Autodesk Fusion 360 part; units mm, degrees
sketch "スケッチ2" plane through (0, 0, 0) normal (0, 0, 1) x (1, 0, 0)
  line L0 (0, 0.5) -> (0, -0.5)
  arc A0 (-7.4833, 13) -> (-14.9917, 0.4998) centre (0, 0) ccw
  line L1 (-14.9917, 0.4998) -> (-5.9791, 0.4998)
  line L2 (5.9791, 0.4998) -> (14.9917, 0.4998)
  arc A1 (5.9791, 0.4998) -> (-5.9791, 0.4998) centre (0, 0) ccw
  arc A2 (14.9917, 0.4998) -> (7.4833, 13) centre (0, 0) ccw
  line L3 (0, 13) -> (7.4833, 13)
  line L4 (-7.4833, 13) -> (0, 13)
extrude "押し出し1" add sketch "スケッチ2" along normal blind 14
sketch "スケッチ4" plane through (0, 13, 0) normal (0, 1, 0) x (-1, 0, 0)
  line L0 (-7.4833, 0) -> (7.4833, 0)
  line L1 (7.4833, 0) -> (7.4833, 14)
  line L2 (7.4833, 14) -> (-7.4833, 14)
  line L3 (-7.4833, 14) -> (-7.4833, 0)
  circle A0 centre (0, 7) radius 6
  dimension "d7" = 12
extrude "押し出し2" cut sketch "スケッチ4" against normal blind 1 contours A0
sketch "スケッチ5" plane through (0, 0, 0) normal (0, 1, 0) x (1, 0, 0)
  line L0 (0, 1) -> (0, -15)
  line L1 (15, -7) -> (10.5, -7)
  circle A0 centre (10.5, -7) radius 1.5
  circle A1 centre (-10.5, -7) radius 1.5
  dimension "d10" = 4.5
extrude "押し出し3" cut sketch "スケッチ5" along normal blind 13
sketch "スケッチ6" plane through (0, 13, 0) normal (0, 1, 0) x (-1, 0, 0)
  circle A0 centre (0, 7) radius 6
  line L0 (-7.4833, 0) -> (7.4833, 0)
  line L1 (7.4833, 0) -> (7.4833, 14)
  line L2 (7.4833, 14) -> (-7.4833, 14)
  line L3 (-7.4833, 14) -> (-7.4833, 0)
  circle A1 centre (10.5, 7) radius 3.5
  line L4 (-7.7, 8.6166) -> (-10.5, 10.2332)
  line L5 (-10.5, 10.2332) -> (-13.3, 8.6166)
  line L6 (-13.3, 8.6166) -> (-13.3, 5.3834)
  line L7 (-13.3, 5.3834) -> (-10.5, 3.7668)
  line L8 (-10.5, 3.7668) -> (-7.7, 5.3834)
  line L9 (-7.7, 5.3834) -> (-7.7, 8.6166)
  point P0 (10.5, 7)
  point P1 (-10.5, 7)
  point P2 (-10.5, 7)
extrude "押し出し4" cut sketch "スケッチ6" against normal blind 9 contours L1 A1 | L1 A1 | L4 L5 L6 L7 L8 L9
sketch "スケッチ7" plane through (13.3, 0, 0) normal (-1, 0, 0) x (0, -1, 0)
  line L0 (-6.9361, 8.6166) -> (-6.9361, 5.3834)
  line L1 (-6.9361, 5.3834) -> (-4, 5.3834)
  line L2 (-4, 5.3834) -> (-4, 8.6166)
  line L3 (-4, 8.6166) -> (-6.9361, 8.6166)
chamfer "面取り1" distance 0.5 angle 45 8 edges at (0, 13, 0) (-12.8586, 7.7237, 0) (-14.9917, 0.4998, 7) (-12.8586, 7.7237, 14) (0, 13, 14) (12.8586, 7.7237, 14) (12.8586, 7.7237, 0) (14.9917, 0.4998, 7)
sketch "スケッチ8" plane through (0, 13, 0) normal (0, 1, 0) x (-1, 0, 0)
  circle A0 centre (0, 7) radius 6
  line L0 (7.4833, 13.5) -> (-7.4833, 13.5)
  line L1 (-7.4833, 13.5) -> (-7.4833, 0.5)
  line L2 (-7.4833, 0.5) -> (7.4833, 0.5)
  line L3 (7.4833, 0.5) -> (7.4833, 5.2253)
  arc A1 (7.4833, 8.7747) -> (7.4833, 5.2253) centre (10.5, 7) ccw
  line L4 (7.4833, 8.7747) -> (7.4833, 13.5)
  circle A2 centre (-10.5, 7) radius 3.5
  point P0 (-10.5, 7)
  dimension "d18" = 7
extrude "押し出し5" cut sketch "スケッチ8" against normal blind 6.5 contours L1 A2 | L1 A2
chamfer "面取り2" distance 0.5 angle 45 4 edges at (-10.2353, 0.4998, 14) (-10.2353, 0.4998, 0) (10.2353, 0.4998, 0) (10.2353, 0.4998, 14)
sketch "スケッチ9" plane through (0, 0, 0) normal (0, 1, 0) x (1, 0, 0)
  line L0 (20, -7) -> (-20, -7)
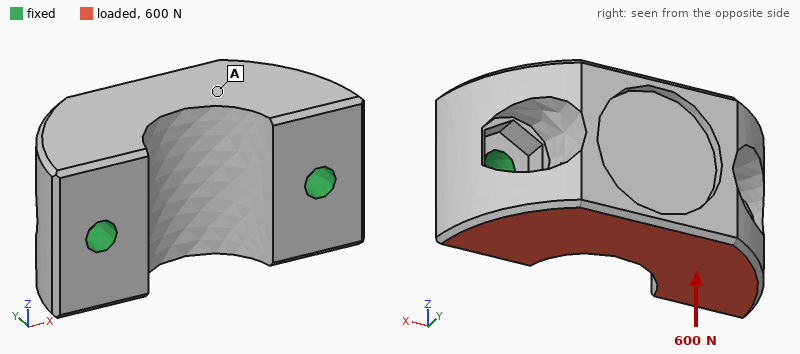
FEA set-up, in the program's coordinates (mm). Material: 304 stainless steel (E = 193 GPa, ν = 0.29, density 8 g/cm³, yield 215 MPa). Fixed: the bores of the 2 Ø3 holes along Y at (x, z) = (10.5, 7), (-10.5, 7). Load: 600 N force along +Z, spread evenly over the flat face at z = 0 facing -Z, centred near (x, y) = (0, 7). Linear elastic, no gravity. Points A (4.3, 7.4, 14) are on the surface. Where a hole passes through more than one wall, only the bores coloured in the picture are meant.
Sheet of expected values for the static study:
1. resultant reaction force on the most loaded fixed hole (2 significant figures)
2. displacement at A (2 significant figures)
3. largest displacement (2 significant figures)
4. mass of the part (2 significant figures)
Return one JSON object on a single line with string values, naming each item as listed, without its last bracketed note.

{"resultant reaction force on the most loaded fixed hole": "300 N", "displacement at A": "2.6 µm", "largest displacement": "4.1 µm", "mass of the part": "25 g"}
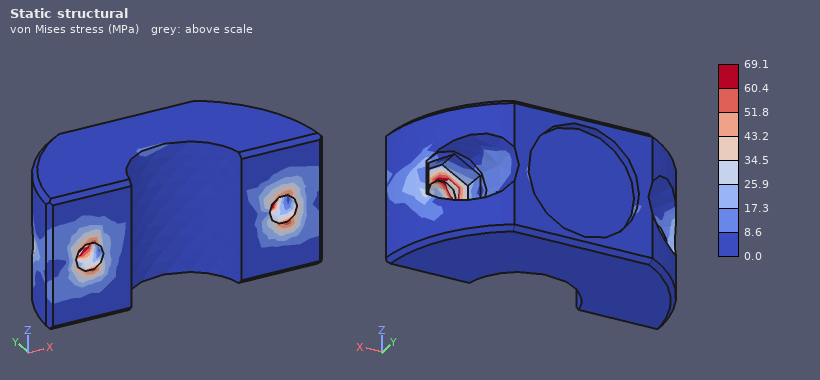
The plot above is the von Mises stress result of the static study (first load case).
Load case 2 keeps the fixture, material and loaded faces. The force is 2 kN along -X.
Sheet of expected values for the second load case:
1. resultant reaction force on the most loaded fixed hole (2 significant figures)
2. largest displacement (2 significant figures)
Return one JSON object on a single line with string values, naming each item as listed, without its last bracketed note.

{"resultant reaction force on the most loaded fixed hole": "1.2 kN", "largest displacement": "4.6 µm"}
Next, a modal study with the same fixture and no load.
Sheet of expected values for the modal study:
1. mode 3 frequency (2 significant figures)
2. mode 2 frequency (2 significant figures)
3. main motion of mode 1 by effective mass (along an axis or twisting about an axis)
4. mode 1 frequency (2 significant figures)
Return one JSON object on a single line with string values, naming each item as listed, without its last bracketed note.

{"mode 3 frequency": "36 kHz", "mode 2 frequency": "36 kHz", "main motion of mode 1 by effective mass": "along Z", "mode 1 frequency": "14 kHz"}
